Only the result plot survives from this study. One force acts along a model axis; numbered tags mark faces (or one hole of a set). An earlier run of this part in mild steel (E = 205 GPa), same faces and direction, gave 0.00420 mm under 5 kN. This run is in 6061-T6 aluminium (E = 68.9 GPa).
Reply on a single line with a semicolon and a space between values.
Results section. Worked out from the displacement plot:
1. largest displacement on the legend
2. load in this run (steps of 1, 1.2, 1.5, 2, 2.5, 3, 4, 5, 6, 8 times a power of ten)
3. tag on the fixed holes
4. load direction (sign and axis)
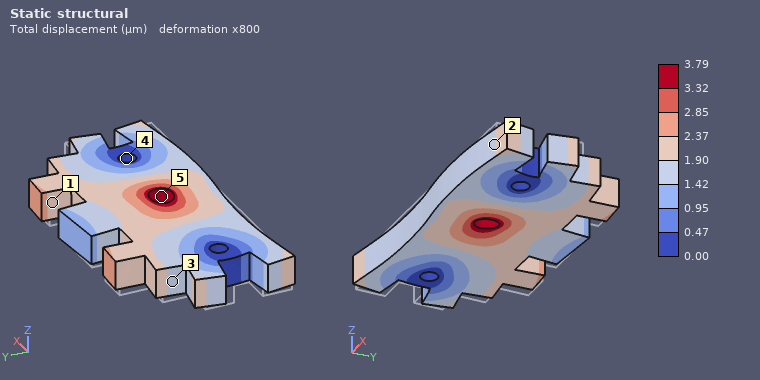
3.79 µm; 1.5 kN; 4; +X
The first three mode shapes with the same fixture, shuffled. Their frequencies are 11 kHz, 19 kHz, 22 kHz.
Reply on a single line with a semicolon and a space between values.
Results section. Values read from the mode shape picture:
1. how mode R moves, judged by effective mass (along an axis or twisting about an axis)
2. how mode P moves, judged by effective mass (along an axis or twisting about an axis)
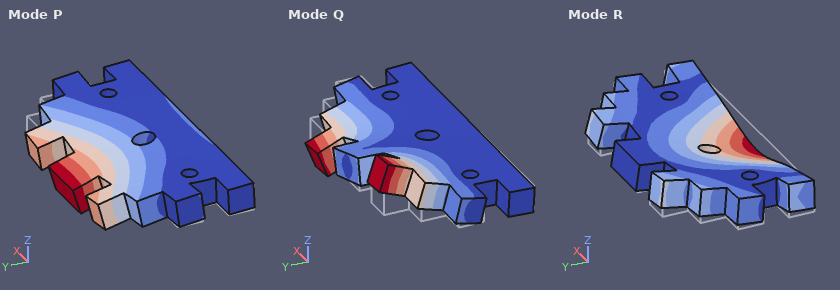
along Z; along Z
